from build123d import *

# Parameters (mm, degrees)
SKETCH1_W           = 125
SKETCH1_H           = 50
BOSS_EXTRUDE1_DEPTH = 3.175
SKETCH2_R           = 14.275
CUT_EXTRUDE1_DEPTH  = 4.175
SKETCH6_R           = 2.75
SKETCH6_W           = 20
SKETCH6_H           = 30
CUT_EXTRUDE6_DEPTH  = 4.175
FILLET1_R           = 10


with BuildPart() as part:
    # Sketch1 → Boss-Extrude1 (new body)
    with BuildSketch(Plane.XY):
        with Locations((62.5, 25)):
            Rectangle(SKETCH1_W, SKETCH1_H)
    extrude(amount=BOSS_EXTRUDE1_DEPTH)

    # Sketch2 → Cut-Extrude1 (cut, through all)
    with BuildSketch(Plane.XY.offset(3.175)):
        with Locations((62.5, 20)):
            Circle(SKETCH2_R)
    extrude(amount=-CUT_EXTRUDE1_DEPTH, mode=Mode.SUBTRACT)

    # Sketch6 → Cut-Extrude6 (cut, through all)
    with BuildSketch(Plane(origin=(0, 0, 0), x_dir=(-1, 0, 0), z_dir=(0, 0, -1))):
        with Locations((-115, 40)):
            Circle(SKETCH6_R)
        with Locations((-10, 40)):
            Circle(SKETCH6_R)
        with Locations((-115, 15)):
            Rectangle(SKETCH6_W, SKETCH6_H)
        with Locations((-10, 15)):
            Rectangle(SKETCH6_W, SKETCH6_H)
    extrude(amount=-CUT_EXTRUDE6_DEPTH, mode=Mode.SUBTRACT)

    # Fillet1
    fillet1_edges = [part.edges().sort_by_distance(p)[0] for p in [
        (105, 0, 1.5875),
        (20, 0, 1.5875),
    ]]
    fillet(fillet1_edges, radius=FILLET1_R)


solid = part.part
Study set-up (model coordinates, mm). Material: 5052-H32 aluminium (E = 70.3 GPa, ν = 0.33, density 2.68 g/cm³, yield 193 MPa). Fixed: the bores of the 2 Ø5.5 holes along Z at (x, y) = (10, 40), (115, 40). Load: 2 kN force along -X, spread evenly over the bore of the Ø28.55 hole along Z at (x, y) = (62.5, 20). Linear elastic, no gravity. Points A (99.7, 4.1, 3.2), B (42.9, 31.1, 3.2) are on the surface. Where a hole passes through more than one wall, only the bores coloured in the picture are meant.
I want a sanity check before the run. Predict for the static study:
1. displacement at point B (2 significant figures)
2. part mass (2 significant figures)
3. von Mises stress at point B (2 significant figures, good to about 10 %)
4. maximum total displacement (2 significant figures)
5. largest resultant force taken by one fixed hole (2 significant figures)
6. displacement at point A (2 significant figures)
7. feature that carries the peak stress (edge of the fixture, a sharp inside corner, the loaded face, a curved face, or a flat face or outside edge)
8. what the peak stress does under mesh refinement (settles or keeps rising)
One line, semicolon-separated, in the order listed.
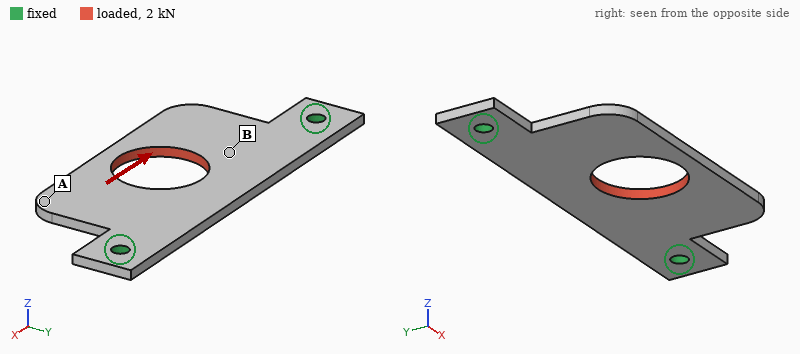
8.0 µm; 37 g; 9.3 MPa; 24 µm; 1.1 kN; 20 µm; a sharp inside corner; keeps rising
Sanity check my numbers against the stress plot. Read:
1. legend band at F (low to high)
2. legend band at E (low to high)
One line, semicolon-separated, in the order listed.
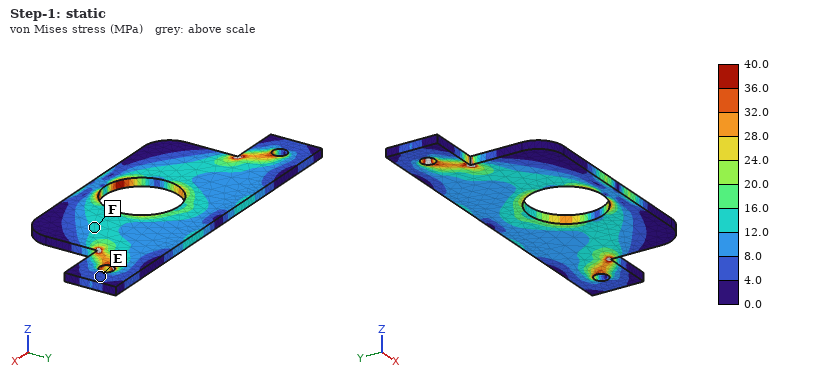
12.0 to 16.0 MPa; 4.0 to 8.0 MPa
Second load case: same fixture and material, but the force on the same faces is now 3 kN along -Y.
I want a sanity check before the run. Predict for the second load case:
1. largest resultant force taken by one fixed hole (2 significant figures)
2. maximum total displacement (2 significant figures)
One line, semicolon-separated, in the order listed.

1.7 kN; 65 µm
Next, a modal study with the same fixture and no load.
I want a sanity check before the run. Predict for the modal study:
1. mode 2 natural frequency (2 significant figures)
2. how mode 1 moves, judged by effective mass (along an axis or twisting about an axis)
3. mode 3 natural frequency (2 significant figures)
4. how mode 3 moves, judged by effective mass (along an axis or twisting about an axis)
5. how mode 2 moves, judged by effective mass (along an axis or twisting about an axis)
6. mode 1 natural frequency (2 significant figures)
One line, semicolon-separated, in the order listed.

1800 Hz; along Z; 2000 Hz; twisting about Y; along Z; 880 Hz
